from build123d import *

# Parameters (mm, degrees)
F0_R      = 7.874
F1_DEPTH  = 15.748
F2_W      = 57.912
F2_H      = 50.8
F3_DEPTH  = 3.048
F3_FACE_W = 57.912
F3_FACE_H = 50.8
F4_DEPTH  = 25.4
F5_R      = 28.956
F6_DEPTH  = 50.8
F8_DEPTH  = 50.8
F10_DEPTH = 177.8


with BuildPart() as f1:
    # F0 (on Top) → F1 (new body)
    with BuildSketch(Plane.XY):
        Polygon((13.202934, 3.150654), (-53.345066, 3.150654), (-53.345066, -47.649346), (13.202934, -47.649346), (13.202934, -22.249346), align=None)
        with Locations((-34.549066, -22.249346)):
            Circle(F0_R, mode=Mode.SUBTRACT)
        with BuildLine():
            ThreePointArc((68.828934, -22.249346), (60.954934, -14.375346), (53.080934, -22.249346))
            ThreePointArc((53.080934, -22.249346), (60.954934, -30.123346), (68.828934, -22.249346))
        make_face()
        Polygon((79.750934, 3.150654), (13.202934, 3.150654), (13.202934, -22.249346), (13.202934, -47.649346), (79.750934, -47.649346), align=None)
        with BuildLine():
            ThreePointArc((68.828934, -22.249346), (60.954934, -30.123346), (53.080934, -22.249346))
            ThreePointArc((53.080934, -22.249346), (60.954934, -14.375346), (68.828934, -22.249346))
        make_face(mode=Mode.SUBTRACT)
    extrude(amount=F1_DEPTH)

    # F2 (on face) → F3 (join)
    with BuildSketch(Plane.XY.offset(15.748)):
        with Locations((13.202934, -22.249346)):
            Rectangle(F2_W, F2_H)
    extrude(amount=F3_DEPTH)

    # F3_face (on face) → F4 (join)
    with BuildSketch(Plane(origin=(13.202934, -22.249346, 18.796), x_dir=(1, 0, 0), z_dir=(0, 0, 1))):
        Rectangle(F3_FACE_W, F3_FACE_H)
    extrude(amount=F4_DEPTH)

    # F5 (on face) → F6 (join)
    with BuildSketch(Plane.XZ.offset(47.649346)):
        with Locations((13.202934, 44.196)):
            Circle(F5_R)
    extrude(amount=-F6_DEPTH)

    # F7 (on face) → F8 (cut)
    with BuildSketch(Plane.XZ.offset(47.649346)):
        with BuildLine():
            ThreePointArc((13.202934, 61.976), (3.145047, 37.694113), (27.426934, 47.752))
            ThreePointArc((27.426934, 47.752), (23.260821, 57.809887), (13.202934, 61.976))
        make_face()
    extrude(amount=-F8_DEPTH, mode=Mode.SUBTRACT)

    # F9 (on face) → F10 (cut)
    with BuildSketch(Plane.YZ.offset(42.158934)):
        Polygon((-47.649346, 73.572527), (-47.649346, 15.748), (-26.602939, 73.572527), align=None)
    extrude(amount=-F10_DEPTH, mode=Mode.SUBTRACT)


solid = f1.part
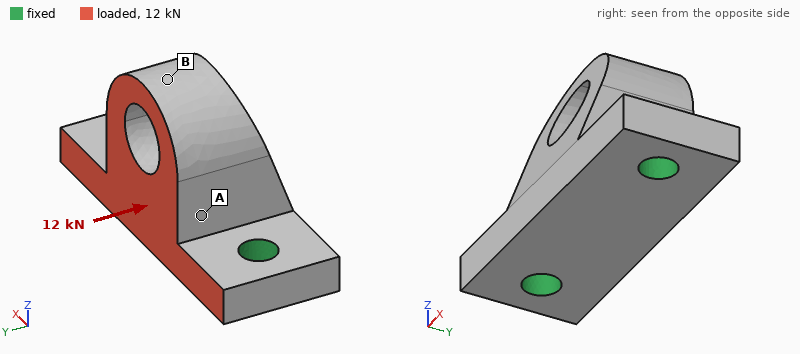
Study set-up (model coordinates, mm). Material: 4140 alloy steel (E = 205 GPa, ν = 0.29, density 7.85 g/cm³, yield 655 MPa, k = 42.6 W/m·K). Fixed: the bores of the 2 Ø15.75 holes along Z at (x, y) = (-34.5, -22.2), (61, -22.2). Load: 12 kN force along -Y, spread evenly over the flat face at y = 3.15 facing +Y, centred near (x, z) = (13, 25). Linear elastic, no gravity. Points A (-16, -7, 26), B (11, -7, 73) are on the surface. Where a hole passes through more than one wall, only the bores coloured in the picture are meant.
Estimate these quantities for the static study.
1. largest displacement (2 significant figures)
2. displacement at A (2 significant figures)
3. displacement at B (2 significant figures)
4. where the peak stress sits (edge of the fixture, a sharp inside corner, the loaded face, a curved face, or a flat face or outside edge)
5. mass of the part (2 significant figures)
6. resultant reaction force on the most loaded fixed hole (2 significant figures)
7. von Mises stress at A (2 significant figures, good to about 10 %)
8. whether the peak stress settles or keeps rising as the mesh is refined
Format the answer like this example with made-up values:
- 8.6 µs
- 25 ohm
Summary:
- 33 µm
- 11 µm
- 32 µm
- edge of the fixture
- 1.6 kg
- 6.0 kN
- 12 MPa
- keeps rising
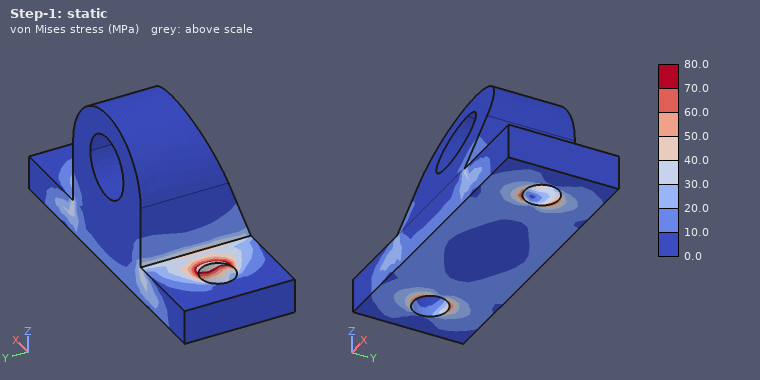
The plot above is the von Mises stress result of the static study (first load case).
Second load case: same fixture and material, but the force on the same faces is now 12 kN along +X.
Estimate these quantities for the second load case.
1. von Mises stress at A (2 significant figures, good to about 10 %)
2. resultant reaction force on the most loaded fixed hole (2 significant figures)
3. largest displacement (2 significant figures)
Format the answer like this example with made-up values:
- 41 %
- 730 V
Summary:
- 10.0 MPa
- 7.2 kN
- 10 µm
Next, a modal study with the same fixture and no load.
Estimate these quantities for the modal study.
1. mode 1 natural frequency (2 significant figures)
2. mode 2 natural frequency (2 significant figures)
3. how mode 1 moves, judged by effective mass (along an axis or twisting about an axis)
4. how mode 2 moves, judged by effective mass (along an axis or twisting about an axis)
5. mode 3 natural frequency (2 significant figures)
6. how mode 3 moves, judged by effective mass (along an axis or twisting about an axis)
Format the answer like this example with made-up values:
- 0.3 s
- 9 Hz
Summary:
- 3200 Hz
- 6600 Hz
- along Y
- along X
- 7100 Hz
- along Z
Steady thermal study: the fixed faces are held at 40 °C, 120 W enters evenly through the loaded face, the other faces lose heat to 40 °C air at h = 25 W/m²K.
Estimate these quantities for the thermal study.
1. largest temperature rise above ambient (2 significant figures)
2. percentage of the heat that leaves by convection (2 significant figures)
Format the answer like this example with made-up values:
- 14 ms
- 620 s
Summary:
- 58 K
- 14 %
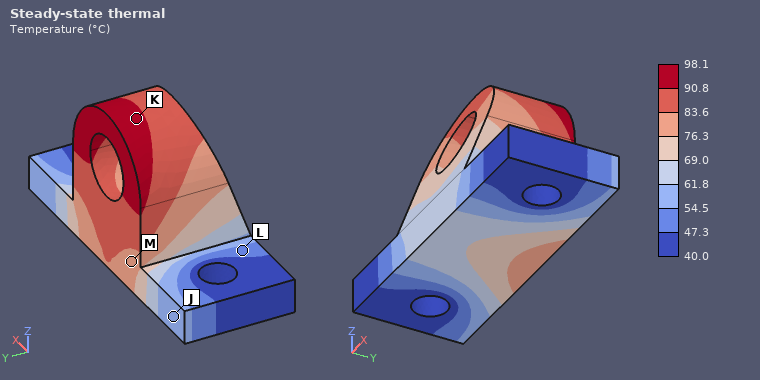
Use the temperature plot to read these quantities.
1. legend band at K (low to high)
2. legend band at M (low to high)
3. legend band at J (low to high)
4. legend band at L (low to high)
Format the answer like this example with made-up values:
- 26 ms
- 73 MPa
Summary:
- 90.8 to 98.1 °C
- 76.3 to 83.6 °C
- 54.5 to 61.8 °C
- 47.3 to 54.5 °C
